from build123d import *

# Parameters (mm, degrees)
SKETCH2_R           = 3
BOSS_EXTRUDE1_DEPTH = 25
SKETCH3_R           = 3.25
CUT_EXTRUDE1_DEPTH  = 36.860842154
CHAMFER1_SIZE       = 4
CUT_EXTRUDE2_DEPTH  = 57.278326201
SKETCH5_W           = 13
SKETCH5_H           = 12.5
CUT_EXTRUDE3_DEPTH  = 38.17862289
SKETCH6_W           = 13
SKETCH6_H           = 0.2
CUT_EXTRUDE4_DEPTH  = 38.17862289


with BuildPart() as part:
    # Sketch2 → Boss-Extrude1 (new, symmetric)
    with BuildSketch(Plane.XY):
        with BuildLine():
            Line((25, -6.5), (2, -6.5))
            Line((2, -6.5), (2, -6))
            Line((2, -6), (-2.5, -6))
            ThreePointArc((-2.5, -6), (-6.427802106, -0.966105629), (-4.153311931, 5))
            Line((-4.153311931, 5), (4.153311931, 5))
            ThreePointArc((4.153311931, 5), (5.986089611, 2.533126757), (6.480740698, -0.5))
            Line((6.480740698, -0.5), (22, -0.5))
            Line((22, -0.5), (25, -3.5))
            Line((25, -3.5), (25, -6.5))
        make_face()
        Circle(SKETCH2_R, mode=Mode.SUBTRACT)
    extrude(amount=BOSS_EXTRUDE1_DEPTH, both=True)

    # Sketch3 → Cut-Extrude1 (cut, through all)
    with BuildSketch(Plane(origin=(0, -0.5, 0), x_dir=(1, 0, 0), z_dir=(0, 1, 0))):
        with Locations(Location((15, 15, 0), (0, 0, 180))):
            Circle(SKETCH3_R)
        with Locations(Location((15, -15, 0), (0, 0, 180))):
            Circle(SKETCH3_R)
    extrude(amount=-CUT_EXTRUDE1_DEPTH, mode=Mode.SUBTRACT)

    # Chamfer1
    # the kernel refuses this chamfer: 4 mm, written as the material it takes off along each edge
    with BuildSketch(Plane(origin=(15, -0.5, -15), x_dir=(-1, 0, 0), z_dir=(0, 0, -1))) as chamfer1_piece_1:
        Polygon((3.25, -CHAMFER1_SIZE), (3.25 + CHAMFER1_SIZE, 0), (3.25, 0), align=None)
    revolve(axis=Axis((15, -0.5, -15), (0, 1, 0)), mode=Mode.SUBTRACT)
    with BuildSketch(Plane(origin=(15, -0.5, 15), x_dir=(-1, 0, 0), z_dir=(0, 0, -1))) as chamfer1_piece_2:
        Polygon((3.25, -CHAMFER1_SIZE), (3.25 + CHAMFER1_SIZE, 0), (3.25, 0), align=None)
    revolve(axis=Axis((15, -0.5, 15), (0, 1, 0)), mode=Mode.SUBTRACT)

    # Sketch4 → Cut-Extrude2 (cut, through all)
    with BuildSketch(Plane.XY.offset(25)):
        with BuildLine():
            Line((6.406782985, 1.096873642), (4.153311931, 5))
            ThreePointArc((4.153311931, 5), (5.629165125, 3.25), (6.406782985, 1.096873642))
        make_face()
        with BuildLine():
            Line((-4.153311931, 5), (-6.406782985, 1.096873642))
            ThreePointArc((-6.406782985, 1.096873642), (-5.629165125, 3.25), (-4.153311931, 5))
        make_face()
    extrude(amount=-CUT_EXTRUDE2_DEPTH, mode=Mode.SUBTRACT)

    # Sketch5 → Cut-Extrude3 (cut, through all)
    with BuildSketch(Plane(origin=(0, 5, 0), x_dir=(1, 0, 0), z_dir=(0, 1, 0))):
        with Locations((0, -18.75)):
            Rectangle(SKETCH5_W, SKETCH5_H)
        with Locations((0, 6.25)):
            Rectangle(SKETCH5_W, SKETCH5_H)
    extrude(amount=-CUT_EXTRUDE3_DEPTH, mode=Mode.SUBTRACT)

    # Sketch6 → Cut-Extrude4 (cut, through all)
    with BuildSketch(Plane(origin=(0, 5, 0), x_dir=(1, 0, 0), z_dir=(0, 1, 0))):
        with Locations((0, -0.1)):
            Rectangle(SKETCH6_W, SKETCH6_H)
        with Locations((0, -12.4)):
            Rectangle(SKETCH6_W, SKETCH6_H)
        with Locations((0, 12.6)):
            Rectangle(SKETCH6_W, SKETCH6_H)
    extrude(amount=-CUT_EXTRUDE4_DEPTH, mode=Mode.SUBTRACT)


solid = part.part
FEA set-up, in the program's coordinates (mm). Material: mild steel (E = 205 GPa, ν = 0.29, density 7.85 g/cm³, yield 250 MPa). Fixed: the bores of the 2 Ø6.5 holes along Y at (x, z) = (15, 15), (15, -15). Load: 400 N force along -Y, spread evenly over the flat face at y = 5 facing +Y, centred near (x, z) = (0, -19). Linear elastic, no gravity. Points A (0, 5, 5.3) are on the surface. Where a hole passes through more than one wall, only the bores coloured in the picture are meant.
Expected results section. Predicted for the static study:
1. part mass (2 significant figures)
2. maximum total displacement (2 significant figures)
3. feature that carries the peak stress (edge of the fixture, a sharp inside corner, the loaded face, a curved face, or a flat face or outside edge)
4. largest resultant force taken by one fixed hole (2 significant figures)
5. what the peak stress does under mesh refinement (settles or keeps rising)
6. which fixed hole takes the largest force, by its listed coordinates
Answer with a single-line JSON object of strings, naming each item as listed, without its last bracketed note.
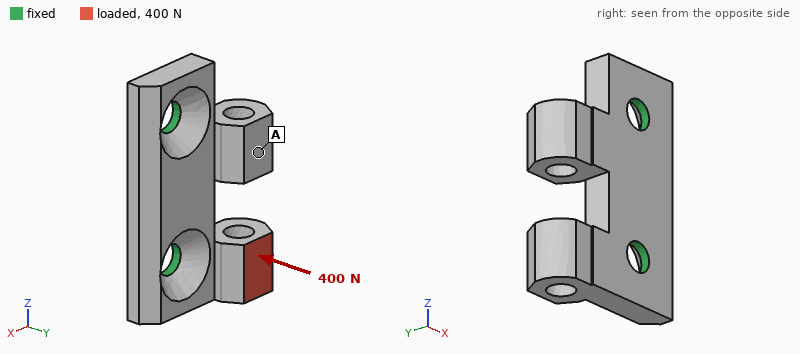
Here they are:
{"part mass": "54 g", "maximum total displacement": "34 µm", "feature that carries the peak stress": "a sharp inside corner", "largest resultant force taken by one fixed hole": "440 N", "what the peak stress does under mesh refinement": "keeps rising", "which fixed hole takes the largest force, by its listed coordinates": "(15, -15)"}
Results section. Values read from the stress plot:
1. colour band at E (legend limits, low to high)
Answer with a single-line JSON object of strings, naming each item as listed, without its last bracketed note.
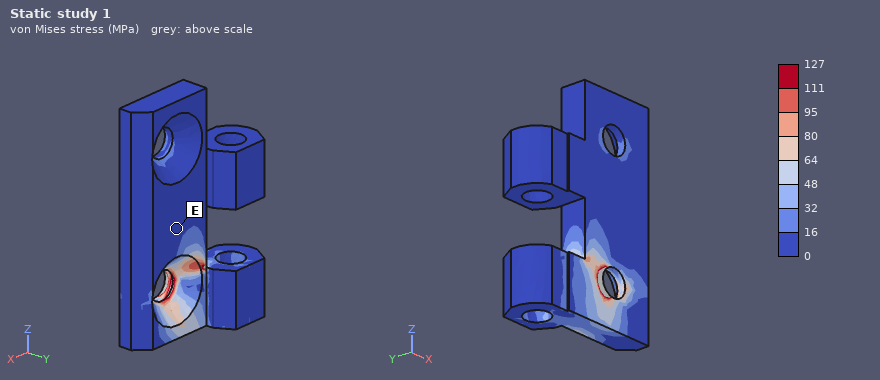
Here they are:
{"colour band at E": "0 to 16 MPa"}
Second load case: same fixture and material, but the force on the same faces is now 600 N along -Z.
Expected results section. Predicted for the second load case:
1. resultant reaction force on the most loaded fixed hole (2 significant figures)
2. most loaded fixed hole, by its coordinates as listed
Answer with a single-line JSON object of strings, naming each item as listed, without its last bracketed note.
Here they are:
{"resultant reaction force on the most loaded fixed hole": "470 N", "most loaded fixed hole, by its coordinates as listed": "(15, 15)"}
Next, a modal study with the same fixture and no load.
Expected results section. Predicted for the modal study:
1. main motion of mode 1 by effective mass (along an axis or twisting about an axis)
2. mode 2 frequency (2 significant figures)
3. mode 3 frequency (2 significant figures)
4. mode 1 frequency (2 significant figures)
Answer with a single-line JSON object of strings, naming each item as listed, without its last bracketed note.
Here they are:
{"main motion of mode 1 by effective mass": "along Y", "mode 2 frequency": "7600 Hz", "mode 3 frequency": "14 kHz", "mode 1 frequency": "6300 Hz"}
